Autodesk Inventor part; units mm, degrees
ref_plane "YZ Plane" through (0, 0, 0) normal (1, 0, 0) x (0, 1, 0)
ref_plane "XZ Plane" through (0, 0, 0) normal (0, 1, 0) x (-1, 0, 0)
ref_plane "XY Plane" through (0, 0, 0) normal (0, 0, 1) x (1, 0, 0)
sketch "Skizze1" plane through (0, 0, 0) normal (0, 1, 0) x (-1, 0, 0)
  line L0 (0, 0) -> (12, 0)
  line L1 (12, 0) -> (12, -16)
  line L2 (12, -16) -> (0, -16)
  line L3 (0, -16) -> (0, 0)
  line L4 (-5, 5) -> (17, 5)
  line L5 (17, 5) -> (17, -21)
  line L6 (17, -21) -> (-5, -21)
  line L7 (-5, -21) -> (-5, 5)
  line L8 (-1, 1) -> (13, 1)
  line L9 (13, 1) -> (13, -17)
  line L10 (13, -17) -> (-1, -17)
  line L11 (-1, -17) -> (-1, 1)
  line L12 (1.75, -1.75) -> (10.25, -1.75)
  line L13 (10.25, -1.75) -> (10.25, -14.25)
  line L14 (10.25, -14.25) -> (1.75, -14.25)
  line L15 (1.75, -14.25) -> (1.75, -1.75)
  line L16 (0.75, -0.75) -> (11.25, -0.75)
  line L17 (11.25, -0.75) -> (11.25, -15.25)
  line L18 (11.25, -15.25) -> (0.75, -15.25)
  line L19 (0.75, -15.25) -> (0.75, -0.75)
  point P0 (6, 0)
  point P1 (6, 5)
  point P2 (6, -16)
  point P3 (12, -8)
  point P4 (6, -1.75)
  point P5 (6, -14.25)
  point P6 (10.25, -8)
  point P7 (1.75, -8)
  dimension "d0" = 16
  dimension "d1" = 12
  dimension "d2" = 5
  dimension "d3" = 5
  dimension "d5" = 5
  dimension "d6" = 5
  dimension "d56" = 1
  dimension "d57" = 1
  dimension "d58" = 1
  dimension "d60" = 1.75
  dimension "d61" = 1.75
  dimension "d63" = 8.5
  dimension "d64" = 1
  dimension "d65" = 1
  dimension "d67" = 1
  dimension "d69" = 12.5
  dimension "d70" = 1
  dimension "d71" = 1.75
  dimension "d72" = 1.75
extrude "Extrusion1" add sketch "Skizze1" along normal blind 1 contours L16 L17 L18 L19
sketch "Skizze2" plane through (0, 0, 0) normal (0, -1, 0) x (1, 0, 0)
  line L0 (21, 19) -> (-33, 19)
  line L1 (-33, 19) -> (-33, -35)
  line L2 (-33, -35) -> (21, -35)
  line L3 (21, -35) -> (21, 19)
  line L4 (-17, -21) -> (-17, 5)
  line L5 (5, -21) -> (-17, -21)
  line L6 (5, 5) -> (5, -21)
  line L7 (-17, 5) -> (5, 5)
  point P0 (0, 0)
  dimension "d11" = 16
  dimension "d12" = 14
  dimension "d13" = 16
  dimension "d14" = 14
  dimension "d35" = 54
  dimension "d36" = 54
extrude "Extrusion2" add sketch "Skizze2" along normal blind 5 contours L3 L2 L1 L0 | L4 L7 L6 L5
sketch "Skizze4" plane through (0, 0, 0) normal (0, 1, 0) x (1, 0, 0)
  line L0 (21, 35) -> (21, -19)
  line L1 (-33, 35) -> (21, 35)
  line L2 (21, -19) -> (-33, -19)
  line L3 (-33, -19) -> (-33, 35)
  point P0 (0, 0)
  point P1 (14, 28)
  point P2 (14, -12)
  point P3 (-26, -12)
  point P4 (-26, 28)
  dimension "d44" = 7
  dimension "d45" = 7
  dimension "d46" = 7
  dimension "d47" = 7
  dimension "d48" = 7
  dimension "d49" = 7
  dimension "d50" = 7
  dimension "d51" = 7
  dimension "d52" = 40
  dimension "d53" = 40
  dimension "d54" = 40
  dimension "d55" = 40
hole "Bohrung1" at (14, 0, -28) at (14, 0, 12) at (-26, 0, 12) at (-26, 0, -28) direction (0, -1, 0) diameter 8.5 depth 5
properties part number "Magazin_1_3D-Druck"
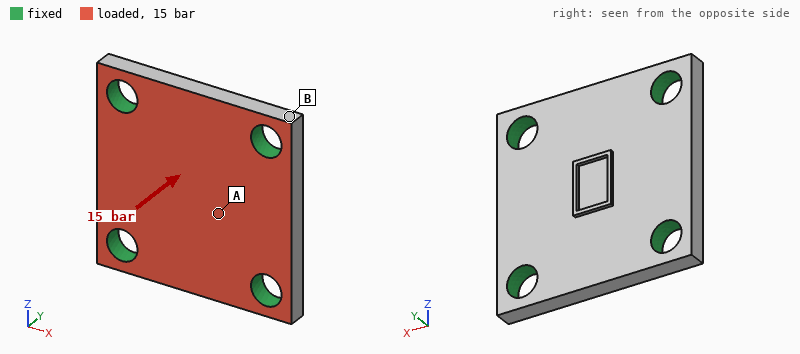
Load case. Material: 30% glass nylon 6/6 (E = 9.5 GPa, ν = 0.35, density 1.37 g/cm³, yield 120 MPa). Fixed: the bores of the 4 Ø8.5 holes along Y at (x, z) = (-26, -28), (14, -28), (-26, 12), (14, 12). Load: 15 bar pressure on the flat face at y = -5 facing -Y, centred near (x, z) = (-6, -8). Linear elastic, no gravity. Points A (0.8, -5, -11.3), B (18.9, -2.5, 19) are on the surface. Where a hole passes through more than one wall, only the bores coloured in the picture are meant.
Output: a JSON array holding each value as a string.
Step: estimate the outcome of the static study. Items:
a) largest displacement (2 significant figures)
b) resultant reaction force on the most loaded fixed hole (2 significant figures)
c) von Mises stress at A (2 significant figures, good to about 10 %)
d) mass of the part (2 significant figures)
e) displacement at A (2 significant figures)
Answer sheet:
["0.16 mm", "1.0 kN", "18 MPa", "18 g", "0.14 mm"]
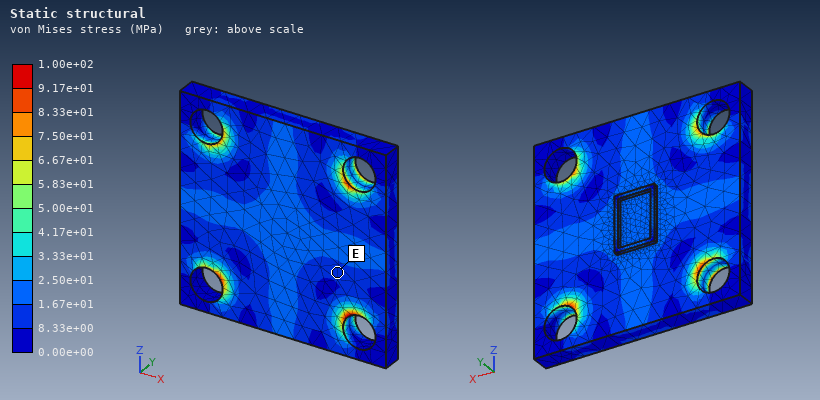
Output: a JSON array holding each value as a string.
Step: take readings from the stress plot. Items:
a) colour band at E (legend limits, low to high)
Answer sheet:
["8.33e+00 to 1.67e+01 MPa"]
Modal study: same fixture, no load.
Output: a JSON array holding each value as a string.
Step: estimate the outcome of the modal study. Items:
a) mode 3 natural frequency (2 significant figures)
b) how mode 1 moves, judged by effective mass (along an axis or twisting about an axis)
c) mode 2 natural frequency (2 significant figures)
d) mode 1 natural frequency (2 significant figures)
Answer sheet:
["11 kHz", "along Y", "11 kHz", "7200 Hz"]
